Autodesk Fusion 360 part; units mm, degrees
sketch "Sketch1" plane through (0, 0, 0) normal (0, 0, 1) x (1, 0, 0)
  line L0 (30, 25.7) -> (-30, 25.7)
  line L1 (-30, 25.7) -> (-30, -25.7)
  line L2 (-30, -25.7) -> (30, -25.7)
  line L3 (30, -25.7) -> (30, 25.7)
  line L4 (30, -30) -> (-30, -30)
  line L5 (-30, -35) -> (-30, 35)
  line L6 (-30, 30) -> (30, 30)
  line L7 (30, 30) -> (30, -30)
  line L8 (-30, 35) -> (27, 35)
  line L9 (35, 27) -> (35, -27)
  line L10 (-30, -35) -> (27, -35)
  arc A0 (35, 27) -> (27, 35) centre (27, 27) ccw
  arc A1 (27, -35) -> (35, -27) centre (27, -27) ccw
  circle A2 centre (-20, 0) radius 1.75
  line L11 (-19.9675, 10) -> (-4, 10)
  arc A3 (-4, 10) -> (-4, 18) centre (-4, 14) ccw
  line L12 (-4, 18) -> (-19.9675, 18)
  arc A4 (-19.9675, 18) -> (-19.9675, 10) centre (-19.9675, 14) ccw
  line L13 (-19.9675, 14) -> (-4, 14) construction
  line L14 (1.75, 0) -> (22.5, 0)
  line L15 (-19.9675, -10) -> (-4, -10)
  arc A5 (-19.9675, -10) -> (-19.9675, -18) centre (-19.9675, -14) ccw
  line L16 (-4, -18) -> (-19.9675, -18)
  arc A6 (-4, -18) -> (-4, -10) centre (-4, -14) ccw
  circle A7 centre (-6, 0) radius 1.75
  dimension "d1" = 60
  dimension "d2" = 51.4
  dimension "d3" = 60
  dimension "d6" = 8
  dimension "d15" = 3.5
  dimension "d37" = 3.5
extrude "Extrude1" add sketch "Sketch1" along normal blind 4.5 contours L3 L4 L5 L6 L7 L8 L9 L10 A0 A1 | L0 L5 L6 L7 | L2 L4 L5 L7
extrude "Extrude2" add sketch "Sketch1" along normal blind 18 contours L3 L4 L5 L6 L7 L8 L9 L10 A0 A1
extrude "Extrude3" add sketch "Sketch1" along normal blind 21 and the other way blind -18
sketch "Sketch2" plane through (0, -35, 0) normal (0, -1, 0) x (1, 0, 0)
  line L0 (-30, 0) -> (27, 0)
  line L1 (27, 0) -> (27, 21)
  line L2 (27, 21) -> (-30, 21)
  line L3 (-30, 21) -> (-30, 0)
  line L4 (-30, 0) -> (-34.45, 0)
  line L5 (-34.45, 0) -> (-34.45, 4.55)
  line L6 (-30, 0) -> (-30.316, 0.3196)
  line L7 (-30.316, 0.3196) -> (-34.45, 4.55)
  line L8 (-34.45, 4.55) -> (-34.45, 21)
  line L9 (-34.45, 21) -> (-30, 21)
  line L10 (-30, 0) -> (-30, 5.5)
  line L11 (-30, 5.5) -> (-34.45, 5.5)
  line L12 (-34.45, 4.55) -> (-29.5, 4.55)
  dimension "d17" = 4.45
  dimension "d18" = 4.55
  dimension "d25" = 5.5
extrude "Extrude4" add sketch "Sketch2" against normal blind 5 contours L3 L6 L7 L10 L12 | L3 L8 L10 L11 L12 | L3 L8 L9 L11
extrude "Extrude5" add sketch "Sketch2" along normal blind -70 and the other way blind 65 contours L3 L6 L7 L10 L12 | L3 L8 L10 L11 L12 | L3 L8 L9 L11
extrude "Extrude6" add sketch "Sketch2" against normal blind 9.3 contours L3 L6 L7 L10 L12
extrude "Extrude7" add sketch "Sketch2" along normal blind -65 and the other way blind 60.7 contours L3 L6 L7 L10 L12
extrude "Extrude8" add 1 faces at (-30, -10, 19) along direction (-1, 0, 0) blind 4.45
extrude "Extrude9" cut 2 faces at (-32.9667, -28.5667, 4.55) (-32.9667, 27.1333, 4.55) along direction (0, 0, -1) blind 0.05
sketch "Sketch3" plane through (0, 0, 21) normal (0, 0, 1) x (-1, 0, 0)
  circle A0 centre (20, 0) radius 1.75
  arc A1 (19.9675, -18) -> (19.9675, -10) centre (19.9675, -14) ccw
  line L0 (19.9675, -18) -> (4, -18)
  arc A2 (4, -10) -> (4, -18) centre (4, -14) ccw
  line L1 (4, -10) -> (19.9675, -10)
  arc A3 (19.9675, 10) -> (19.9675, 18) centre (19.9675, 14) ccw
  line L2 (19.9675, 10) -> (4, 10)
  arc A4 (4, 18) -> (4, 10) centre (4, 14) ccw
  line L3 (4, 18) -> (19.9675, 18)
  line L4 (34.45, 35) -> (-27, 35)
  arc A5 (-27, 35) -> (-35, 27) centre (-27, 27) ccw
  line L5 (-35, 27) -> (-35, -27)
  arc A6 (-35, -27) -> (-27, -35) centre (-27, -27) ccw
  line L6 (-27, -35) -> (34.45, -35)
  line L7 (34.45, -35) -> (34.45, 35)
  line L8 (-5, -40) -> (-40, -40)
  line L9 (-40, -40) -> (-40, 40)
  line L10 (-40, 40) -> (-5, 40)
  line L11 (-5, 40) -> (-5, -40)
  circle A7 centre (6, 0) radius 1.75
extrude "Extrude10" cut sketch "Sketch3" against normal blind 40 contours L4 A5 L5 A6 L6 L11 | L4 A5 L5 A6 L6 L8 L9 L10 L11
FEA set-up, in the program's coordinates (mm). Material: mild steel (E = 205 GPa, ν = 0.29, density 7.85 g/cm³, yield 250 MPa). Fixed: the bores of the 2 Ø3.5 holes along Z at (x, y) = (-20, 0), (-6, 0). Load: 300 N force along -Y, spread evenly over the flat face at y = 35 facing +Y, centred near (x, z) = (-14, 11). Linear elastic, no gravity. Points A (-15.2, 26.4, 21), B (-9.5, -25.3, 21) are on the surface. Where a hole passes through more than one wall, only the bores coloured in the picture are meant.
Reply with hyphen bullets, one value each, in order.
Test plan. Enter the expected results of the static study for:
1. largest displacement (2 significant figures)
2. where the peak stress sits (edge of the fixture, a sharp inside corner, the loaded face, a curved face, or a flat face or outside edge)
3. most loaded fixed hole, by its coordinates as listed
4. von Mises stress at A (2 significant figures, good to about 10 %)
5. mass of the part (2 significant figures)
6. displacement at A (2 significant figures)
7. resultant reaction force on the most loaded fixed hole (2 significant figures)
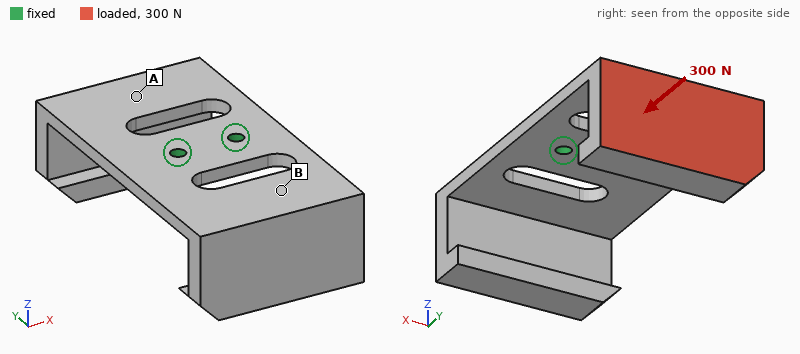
- 0.22 mm
- a curved face
- (-20, 0)
- 29 MPa
- 120 g
- 0.095 mm
- 180 N
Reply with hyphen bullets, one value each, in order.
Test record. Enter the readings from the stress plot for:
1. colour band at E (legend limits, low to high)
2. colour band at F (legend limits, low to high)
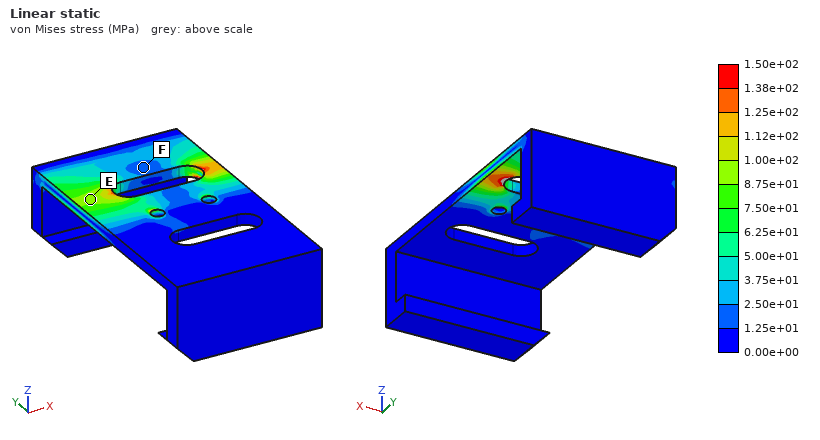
- 8.75e+01 to 1.00e+02 MPa
- 1.25e+01 to 2.50e+01 MPa
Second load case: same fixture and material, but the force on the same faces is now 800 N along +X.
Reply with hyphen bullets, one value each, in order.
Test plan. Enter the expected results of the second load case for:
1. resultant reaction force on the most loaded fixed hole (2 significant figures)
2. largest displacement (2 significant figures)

- 1.7 kN
- 0.18 mm
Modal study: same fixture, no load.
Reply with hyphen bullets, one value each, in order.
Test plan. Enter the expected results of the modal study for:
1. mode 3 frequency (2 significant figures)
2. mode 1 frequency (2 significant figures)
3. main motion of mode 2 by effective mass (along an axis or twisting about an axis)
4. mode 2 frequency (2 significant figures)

- 1500 Hz
- 630 Hz
- along Z
- 680 Hz
